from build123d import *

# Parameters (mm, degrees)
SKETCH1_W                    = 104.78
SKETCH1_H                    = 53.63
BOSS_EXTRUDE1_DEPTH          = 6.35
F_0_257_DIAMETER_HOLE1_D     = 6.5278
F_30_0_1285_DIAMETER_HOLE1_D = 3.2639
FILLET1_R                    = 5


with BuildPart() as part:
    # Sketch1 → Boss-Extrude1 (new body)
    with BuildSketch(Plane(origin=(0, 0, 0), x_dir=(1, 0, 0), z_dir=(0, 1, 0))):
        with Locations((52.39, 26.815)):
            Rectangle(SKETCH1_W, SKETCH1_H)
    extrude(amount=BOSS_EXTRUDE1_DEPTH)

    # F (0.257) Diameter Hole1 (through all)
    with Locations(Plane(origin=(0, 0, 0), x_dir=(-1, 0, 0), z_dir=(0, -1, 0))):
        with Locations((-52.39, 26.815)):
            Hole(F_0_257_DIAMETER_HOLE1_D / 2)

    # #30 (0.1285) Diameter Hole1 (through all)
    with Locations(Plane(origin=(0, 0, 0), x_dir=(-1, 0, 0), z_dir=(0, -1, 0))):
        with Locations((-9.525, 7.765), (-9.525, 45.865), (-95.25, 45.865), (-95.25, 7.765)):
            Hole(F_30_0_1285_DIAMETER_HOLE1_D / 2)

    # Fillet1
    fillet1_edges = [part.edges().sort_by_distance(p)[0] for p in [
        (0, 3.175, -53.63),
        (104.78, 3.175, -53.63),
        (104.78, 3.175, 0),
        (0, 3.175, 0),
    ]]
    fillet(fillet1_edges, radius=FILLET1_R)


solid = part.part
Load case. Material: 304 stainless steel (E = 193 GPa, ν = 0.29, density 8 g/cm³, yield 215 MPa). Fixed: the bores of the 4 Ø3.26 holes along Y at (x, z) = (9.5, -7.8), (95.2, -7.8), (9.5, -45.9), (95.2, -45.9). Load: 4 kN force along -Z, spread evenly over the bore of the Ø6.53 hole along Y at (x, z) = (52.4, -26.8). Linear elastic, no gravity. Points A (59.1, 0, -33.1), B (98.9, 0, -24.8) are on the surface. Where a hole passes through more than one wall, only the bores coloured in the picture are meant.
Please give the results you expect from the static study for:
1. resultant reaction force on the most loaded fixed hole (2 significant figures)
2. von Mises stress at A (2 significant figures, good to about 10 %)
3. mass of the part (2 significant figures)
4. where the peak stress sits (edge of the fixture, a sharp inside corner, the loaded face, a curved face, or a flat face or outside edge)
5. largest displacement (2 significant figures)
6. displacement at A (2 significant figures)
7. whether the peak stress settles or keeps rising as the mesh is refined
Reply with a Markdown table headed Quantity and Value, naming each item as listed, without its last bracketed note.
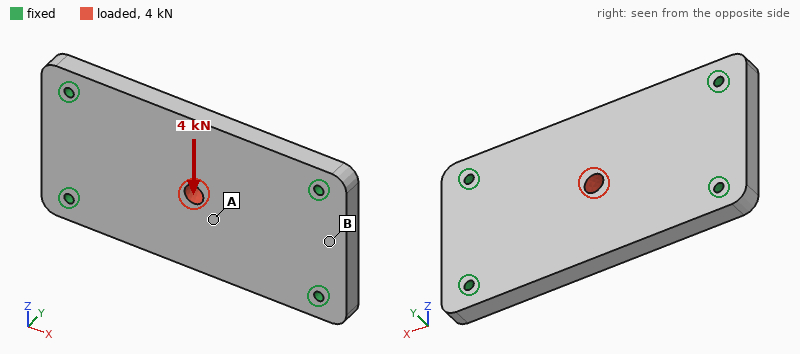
| Quantity | Value |
|---|---|
| resultant reaction force on the most loaded fixed hole | 1.4 kN |
| von Mises stress at A | 17 MPa |
| mass of the part | 280 g |
| where the peak stress sits | edge of the fixture |
| largest displacement | 5.8 µm |
| displacement at A | 4.7 µm |
| whether the peak stress settles or keeps rising as the mesh is refined | keeps rising |
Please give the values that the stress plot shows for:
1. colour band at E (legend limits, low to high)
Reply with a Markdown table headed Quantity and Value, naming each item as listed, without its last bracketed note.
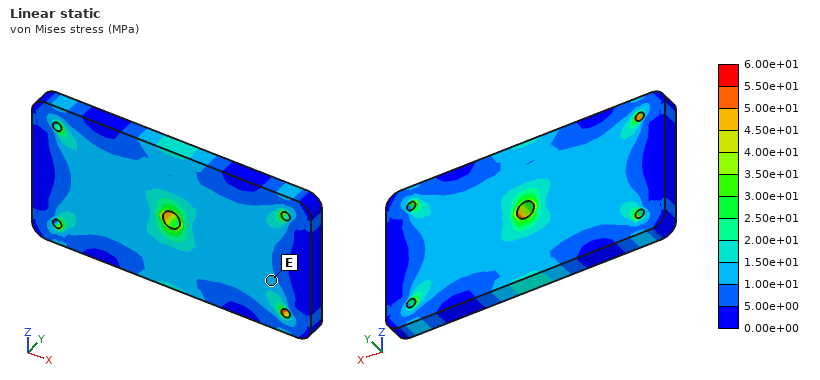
| Quantity | Value |
|---|---|
| colour band at E | 1.00e+01 to 1.50e+01 MPa |
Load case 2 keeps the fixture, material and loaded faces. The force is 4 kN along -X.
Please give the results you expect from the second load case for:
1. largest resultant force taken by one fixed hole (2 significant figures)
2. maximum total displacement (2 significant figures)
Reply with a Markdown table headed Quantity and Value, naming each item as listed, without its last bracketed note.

| Quantity | Value |
|---|---|
| largest resultant force taken by one fixed hole | 1.0 kN |
| maximum total displacement | 2.9 µm |
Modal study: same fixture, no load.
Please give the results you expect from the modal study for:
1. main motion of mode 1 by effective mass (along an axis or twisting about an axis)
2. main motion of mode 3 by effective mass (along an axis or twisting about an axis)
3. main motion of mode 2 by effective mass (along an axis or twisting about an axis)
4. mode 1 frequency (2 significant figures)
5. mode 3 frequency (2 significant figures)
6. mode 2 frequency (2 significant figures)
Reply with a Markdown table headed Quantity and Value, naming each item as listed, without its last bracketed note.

| Quantity | Value |
|---|---|
| main motion of mode 1 by effective mass | along Y |
| main motion of mode 3 by effective mass | twisting about Z |
| main motion of mode 2 by effective mass | twisting about X |
| mode 1 frequency | 3700 Hz |
| mode 3 frequency | 9800 Hz |
| mode 2 frequency | 5800 Hz |
